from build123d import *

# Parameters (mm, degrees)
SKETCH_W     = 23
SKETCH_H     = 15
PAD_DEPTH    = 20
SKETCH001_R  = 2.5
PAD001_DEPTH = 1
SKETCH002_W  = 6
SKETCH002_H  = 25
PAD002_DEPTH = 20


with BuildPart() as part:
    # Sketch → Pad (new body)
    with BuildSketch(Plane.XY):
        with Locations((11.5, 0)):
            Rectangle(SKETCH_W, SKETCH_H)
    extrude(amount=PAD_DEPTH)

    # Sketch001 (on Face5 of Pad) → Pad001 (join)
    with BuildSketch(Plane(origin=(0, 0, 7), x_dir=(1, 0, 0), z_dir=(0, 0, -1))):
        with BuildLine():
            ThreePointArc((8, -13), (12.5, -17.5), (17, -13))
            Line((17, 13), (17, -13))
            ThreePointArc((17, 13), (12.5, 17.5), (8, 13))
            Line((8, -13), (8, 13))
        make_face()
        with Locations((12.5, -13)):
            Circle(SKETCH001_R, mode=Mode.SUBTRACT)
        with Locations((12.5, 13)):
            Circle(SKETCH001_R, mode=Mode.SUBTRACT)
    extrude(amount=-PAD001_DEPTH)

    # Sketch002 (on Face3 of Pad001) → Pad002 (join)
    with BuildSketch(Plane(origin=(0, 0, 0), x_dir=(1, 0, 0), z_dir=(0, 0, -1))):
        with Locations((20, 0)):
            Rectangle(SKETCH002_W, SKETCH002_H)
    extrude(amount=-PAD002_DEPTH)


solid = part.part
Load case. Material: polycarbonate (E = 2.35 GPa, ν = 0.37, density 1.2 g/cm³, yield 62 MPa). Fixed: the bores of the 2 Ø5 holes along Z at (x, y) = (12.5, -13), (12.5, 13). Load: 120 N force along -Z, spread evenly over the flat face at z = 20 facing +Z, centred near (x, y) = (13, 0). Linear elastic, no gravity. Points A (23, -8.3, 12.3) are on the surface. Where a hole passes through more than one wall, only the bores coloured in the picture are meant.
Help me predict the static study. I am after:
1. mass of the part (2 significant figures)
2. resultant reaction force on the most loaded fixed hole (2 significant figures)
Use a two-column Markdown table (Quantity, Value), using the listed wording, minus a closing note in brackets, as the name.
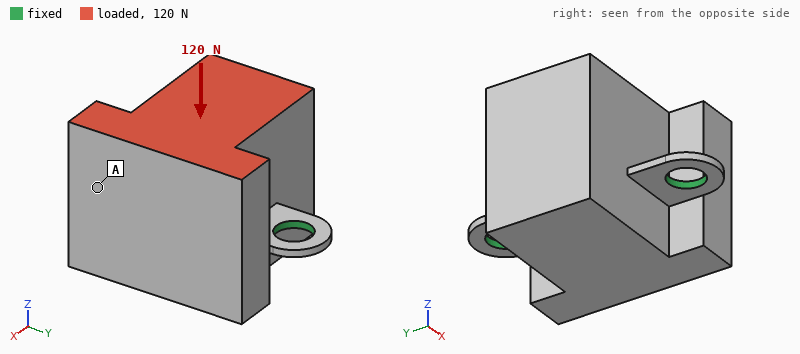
| Quantity | Value |
|---|---|
| mass of the part | 9.9 g |
| resultant reaction force on the most loaded fixed hole | 60 N |
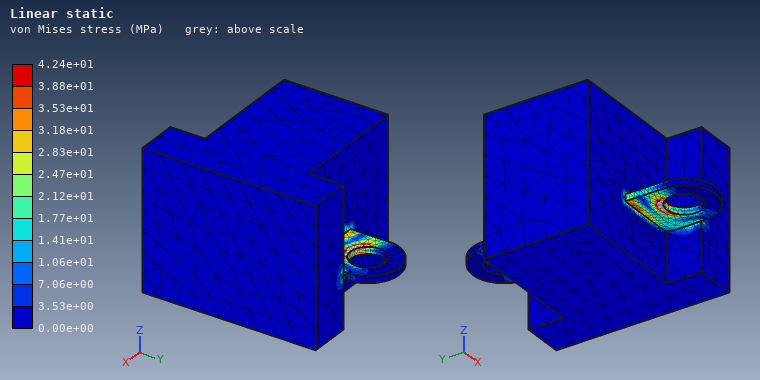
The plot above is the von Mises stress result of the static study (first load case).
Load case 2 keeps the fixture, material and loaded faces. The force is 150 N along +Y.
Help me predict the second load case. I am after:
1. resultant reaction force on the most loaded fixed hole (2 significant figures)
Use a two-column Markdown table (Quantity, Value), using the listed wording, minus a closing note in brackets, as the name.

| Quantity | Value |
|---|---|
| resultant reaction force on the most loaded fixed hole | 120 N |
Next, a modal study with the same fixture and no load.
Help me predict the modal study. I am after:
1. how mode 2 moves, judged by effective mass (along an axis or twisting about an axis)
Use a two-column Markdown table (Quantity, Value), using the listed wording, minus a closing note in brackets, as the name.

| Quantity | Value |
|---|---|
| how mode 2 moves, judged by effective mass | along Z |
